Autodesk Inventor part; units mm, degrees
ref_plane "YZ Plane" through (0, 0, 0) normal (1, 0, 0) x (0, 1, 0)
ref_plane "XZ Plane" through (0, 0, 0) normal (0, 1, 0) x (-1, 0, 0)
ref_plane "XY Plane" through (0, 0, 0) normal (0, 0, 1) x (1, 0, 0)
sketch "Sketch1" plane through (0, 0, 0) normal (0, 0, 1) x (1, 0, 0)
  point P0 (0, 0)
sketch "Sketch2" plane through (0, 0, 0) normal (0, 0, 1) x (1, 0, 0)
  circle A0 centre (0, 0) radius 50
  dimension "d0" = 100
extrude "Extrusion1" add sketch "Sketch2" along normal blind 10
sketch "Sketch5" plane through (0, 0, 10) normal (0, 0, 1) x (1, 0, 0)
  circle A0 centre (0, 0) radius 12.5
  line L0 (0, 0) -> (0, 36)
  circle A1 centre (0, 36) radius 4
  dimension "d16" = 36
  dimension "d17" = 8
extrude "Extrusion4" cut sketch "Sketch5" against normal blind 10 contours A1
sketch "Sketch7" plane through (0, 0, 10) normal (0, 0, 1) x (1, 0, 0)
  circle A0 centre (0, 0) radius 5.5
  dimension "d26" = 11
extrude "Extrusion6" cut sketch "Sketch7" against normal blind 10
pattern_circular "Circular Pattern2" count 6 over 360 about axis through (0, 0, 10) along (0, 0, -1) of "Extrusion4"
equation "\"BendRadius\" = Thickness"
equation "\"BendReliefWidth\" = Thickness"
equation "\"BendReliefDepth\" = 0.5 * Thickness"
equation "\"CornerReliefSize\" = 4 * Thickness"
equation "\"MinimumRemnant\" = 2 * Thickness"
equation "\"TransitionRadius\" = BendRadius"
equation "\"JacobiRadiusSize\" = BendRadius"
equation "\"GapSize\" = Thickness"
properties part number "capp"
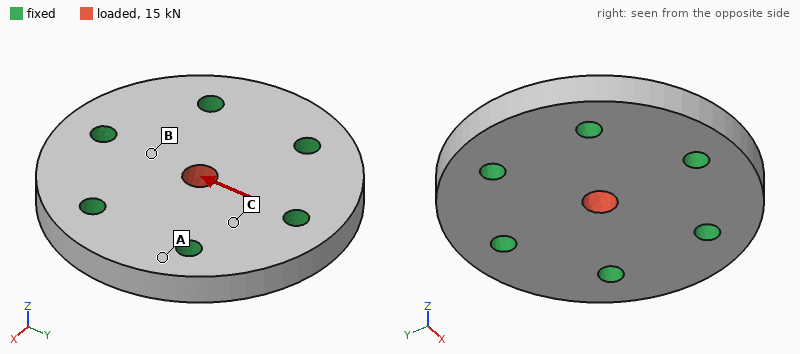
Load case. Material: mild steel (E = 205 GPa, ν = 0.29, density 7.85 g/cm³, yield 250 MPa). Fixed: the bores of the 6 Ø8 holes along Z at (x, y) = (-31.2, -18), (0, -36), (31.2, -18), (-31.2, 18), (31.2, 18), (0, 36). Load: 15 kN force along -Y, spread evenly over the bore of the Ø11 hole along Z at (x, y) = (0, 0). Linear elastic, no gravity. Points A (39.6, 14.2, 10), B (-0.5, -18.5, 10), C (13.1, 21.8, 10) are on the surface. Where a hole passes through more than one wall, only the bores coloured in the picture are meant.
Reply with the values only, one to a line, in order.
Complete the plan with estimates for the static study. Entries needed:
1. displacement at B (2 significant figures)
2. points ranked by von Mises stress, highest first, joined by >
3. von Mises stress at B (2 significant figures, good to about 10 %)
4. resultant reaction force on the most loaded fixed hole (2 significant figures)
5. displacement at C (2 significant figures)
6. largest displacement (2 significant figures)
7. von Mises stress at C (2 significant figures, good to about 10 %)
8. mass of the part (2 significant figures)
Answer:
1.7 µm
B > C > A
26 MPa
4.0 kN
1.1 µm
3.8 µm
9.5 MPa
590 g
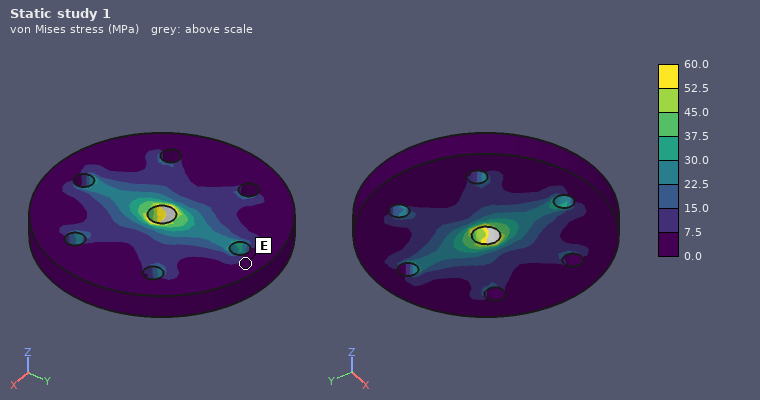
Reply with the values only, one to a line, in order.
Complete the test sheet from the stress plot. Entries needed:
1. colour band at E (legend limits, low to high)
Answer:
0.0 to 7.5 MPa
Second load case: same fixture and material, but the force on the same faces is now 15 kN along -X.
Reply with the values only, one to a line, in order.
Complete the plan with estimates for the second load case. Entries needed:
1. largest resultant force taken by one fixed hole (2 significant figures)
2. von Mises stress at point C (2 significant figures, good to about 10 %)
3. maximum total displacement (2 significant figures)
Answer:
3.5 kN
7.4 MPa
3.8 µm
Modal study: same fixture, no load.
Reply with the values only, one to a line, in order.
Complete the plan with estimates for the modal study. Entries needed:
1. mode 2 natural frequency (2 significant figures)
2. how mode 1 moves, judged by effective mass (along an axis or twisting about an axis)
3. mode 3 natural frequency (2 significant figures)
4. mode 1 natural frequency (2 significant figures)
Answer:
21 kHz
along Z
21 kHz
16 kHz
